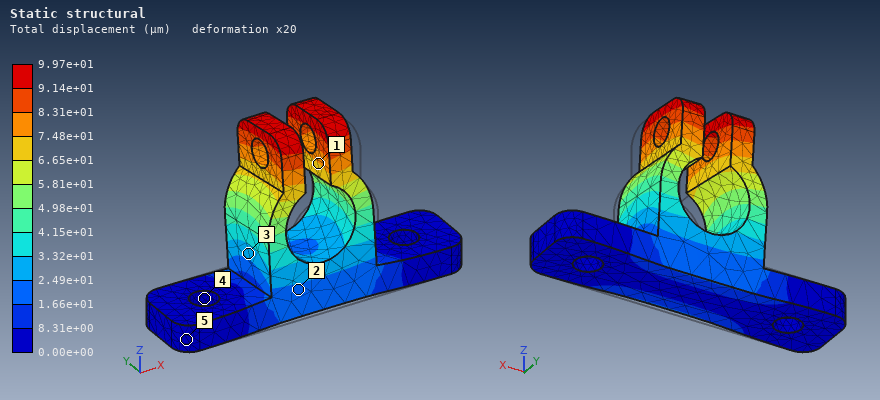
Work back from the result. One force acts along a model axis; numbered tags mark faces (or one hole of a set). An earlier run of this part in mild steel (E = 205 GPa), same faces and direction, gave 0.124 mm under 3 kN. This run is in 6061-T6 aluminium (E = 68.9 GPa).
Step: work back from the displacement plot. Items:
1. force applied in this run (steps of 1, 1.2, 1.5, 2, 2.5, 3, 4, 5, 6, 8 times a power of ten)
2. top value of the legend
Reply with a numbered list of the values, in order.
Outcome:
1. 800 N
2. 9.97e+01 µm
